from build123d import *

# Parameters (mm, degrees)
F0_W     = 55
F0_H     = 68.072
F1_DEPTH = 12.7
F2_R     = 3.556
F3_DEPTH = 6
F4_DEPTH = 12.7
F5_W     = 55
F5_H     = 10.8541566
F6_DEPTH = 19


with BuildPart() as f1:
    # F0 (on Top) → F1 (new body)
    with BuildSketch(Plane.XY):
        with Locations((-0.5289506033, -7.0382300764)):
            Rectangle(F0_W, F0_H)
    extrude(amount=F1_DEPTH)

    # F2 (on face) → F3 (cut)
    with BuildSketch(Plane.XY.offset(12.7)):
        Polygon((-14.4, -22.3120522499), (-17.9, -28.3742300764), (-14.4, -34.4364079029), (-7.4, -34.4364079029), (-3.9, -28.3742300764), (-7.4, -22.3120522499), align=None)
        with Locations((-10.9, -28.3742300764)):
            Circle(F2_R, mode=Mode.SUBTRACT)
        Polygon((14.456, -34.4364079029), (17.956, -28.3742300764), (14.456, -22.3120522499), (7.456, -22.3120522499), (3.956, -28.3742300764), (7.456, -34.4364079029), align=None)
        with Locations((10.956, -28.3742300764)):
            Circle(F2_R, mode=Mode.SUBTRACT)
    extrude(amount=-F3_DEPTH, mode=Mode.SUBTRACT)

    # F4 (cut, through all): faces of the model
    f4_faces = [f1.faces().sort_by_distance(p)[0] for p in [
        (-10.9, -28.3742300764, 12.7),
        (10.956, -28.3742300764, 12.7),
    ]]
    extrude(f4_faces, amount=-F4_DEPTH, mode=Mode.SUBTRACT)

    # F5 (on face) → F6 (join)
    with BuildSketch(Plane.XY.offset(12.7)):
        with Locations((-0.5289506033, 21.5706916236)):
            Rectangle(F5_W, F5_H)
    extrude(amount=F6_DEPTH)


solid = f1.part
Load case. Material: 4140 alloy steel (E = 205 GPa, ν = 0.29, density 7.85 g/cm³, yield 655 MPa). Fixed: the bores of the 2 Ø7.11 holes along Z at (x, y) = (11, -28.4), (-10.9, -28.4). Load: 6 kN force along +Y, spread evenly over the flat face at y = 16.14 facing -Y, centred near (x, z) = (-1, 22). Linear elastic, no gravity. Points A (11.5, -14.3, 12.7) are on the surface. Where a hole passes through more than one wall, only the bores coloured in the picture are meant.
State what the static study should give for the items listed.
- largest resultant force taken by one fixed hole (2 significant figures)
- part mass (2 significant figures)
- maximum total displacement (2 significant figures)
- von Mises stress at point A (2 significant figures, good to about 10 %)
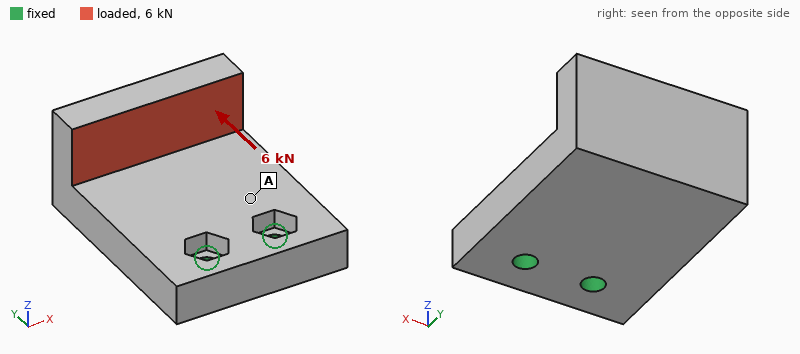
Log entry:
3.1 kN
450 g
0.17 mm
54 MPa
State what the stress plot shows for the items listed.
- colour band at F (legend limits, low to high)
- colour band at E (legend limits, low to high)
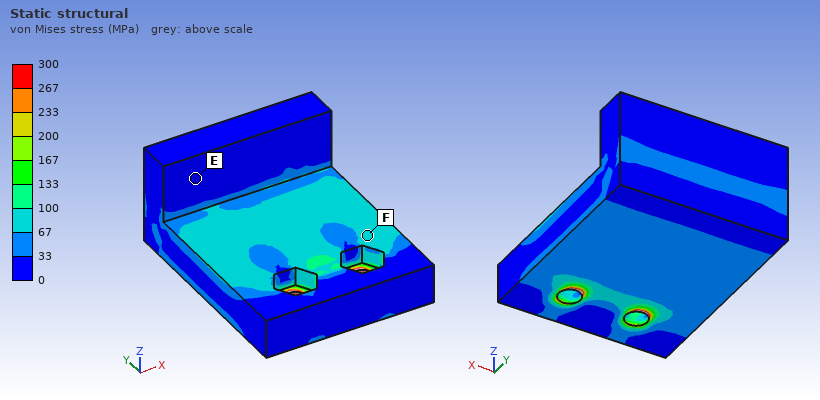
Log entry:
67 to 100 MPa
0 to 33 MPa
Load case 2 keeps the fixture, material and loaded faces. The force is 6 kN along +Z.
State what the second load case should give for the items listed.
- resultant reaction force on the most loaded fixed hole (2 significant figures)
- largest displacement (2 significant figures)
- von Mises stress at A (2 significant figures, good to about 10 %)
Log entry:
3.2 kN
0.28 mm
86 MPa
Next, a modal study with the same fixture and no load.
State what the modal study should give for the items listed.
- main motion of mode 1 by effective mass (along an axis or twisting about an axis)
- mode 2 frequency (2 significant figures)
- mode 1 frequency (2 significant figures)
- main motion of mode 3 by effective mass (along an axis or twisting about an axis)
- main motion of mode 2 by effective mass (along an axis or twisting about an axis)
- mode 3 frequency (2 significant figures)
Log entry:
along Z
4000 Hz
1700 Hz
along X
along X
5200 Hz
